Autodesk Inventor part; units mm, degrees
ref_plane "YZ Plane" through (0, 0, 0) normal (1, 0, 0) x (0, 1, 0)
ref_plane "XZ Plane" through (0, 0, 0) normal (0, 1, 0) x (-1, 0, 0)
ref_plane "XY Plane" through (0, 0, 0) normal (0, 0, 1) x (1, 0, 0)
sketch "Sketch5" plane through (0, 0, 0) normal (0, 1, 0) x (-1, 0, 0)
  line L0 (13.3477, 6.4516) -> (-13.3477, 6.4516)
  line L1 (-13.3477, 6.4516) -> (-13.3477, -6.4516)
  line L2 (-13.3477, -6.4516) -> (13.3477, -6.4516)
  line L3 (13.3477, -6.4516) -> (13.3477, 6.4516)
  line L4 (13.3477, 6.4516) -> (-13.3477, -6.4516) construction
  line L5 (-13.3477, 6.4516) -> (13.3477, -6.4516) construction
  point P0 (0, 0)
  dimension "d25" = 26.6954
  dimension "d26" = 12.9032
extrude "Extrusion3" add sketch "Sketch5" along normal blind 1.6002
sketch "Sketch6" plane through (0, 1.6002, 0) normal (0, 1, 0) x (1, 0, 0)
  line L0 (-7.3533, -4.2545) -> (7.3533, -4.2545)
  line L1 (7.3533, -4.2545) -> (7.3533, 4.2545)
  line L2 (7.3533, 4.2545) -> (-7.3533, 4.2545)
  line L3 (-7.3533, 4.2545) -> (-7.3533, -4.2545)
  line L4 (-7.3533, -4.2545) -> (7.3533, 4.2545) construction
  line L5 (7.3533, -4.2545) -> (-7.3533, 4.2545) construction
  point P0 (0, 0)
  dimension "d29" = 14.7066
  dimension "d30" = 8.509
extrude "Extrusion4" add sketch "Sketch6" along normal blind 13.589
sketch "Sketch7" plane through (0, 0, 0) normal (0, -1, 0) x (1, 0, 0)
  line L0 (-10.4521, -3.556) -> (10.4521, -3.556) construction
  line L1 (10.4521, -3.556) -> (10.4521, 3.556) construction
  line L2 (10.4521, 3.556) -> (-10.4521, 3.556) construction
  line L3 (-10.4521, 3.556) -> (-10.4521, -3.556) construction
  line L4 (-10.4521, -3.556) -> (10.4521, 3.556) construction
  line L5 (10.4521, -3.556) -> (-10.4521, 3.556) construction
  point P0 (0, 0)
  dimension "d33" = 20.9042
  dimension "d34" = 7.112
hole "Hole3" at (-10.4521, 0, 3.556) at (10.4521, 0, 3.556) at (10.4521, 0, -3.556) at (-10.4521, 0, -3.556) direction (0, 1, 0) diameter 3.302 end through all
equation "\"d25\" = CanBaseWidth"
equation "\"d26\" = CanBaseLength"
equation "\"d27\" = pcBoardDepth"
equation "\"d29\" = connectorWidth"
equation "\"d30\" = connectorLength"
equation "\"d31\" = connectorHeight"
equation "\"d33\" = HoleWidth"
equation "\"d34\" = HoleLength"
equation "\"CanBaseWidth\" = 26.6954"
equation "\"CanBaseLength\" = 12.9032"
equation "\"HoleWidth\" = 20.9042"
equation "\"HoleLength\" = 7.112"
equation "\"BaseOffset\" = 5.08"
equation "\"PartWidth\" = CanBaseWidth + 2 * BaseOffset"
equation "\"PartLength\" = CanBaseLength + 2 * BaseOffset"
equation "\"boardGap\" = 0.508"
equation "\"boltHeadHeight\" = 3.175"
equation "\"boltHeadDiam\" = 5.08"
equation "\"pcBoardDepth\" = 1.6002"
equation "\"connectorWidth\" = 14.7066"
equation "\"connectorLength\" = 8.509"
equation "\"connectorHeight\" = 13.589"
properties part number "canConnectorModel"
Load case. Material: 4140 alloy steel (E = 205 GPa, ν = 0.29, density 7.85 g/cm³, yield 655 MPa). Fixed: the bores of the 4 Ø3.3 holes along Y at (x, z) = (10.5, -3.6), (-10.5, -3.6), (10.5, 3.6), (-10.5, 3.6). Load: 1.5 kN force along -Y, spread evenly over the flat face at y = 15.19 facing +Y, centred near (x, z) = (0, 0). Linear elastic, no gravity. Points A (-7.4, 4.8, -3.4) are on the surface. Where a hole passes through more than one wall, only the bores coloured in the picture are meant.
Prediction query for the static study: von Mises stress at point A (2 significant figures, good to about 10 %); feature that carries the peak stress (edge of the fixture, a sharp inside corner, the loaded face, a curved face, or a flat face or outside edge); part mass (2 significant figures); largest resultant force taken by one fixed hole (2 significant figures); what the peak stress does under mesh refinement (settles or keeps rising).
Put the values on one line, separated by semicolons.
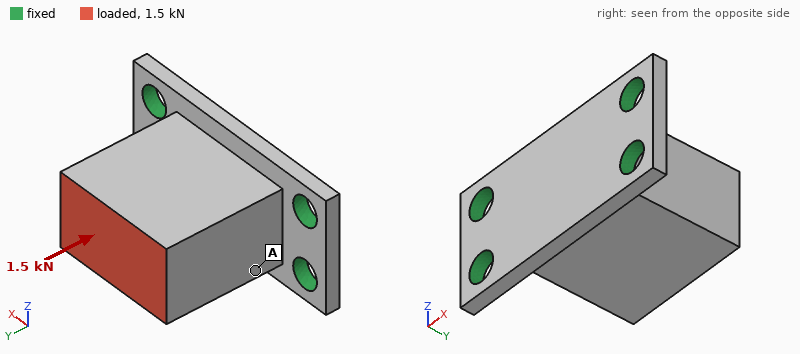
33 MPa; edge of the fixture; 17 g; 420 N; keeps rising
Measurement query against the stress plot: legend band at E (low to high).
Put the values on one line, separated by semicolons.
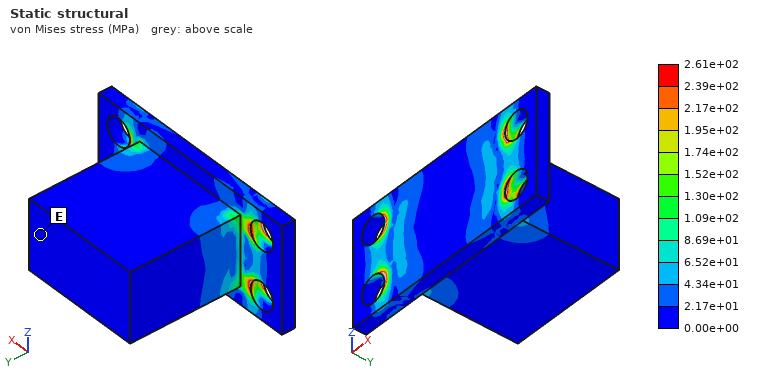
0.00e+00 to 2.17e+01 MPa
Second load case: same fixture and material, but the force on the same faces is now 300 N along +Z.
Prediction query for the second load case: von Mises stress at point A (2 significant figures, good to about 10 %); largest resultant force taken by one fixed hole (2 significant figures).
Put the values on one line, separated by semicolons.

28 MPa; 310 N
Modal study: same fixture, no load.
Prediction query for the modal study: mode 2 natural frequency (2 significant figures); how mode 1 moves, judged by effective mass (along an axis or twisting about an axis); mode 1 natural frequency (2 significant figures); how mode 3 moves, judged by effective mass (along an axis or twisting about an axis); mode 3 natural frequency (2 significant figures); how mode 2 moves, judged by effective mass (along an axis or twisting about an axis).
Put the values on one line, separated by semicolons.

21 kHz; along Z; 9900 Hz; along Y; 24 kHz; along X
